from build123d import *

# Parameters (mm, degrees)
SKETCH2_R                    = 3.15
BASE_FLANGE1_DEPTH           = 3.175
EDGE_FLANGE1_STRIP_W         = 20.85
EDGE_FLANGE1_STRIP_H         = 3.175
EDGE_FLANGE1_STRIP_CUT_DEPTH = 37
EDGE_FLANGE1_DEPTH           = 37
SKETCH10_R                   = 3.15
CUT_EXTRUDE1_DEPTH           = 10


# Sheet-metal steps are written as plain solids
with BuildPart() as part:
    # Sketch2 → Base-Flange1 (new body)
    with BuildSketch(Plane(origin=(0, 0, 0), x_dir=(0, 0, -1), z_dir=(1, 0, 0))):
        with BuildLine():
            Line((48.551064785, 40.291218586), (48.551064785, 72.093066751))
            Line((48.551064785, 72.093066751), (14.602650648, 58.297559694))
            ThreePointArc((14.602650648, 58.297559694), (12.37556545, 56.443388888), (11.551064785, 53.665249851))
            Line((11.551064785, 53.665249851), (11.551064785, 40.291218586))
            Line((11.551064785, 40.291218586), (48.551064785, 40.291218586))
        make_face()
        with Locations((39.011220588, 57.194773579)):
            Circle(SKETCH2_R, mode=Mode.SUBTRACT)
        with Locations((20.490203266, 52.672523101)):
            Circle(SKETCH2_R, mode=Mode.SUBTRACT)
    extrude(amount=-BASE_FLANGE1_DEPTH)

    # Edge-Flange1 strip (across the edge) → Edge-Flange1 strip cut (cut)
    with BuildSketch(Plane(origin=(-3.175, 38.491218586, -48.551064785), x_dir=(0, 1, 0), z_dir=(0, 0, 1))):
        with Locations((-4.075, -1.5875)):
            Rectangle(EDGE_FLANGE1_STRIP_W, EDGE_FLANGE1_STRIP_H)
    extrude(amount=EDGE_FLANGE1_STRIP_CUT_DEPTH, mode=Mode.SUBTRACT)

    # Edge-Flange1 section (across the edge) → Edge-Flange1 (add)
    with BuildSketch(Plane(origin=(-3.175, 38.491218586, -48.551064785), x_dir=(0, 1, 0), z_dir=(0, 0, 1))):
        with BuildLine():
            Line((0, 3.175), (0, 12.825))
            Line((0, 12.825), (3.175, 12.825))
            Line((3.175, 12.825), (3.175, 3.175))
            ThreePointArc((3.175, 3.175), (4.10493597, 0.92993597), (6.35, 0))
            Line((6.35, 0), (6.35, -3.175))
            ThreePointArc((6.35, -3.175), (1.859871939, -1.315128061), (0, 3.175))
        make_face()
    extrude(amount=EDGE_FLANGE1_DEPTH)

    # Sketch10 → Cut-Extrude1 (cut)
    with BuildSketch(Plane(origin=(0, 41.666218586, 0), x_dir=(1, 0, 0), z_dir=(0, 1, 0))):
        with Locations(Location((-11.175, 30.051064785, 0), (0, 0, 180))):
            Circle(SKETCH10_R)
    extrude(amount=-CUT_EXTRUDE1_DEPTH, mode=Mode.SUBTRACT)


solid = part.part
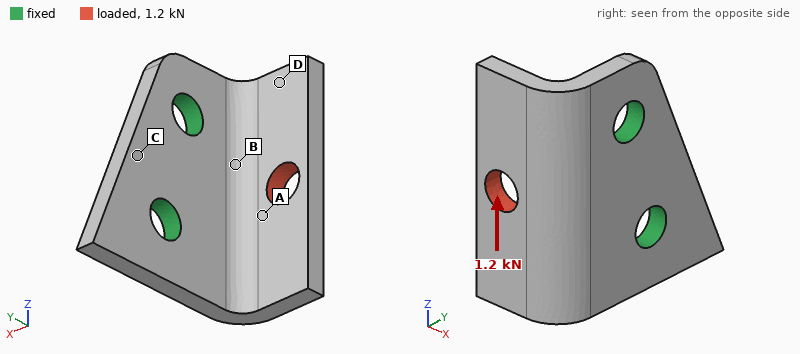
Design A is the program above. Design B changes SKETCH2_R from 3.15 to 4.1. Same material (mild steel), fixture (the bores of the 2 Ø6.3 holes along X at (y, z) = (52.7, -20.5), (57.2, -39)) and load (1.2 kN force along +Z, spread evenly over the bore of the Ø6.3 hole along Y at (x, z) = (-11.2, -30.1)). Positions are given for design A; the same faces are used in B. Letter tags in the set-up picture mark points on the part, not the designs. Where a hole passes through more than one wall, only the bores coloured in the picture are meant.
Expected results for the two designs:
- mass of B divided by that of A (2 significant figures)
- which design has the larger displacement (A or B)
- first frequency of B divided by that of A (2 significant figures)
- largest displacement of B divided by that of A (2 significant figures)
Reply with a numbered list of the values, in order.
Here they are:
1. 0.97
2. A
3. 1.1
4. 0.86
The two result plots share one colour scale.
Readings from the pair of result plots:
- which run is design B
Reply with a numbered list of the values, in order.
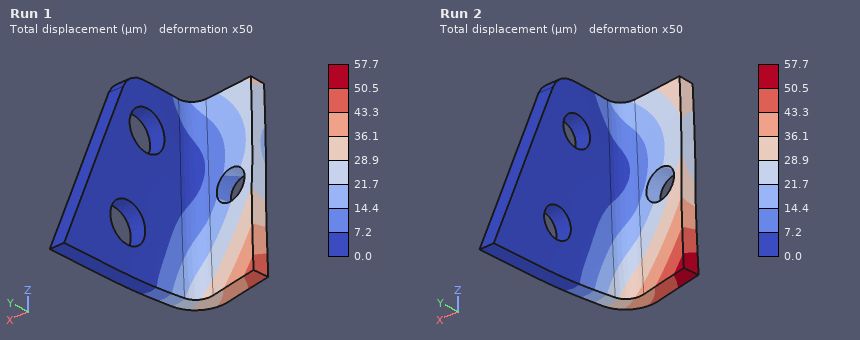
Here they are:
1. Run 1
